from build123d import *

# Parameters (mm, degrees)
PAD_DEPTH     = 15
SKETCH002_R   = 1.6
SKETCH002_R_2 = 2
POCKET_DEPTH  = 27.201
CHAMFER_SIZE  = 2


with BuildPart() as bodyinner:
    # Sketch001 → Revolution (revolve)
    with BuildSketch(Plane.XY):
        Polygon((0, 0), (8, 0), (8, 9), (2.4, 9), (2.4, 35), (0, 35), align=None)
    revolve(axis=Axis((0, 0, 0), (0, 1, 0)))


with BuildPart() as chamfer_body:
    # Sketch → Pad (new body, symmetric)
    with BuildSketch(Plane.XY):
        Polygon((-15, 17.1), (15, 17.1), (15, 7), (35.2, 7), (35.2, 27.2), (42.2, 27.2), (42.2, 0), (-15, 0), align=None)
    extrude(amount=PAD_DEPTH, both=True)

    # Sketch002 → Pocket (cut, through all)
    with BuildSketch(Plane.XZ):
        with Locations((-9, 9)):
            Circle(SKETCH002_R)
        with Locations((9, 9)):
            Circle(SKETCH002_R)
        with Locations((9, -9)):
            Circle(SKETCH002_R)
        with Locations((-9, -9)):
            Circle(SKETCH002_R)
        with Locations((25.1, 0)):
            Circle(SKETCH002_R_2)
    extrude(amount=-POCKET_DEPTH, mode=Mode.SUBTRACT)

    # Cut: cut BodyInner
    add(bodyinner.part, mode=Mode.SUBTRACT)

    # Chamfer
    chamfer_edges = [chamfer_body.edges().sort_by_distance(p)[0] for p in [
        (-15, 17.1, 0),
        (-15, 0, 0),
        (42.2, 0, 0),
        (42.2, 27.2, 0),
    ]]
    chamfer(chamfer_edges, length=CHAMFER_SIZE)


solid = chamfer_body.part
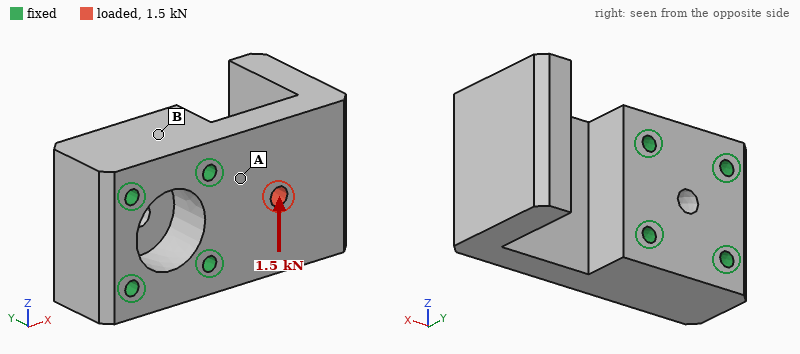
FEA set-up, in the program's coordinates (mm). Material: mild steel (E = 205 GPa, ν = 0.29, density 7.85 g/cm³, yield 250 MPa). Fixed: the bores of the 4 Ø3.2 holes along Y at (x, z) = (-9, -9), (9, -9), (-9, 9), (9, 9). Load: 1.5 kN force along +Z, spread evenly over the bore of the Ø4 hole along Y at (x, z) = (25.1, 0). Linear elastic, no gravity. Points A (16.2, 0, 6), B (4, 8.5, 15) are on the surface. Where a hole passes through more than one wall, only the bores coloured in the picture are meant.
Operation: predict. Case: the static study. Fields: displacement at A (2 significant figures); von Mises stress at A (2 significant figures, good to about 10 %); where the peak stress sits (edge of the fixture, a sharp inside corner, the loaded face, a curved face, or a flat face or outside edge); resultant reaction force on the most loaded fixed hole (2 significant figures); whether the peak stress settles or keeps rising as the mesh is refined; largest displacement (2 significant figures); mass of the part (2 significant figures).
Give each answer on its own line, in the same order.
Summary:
0.78 µm
15 MPa
edge of the fixture
1.3 kN
keeps rising
3.7 µm
180 g
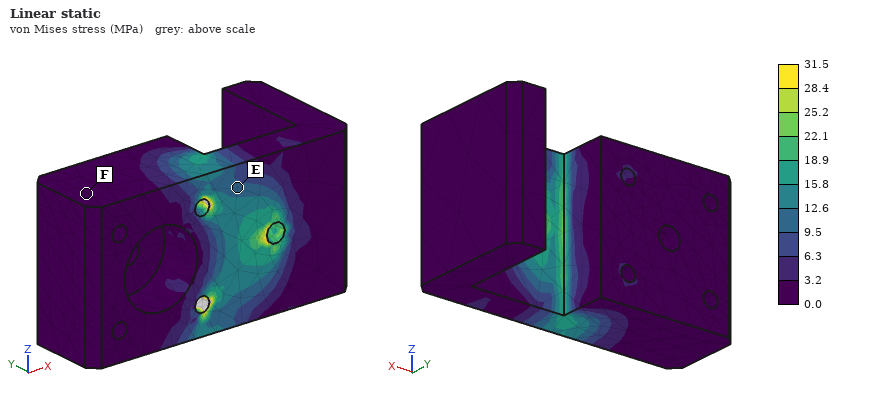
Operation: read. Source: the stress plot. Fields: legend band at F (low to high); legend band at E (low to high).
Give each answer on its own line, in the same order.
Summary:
0.0 to 3.2 MPa
9.5 to 12.6 MPa
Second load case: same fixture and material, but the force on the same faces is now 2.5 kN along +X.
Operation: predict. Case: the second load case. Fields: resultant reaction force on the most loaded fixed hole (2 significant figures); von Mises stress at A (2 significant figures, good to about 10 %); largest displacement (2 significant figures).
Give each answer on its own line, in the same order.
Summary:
1.2 kN
17 MPa
2.1 µm
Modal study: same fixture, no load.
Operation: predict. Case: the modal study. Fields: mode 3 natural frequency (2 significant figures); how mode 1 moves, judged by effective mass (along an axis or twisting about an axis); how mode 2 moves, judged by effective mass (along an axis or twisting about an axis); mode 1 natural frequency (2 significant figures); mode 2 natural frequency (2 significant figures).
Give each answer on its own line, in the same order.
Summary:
8600 Hz
along Y
along Z
2900 Hz
5100 Hz
